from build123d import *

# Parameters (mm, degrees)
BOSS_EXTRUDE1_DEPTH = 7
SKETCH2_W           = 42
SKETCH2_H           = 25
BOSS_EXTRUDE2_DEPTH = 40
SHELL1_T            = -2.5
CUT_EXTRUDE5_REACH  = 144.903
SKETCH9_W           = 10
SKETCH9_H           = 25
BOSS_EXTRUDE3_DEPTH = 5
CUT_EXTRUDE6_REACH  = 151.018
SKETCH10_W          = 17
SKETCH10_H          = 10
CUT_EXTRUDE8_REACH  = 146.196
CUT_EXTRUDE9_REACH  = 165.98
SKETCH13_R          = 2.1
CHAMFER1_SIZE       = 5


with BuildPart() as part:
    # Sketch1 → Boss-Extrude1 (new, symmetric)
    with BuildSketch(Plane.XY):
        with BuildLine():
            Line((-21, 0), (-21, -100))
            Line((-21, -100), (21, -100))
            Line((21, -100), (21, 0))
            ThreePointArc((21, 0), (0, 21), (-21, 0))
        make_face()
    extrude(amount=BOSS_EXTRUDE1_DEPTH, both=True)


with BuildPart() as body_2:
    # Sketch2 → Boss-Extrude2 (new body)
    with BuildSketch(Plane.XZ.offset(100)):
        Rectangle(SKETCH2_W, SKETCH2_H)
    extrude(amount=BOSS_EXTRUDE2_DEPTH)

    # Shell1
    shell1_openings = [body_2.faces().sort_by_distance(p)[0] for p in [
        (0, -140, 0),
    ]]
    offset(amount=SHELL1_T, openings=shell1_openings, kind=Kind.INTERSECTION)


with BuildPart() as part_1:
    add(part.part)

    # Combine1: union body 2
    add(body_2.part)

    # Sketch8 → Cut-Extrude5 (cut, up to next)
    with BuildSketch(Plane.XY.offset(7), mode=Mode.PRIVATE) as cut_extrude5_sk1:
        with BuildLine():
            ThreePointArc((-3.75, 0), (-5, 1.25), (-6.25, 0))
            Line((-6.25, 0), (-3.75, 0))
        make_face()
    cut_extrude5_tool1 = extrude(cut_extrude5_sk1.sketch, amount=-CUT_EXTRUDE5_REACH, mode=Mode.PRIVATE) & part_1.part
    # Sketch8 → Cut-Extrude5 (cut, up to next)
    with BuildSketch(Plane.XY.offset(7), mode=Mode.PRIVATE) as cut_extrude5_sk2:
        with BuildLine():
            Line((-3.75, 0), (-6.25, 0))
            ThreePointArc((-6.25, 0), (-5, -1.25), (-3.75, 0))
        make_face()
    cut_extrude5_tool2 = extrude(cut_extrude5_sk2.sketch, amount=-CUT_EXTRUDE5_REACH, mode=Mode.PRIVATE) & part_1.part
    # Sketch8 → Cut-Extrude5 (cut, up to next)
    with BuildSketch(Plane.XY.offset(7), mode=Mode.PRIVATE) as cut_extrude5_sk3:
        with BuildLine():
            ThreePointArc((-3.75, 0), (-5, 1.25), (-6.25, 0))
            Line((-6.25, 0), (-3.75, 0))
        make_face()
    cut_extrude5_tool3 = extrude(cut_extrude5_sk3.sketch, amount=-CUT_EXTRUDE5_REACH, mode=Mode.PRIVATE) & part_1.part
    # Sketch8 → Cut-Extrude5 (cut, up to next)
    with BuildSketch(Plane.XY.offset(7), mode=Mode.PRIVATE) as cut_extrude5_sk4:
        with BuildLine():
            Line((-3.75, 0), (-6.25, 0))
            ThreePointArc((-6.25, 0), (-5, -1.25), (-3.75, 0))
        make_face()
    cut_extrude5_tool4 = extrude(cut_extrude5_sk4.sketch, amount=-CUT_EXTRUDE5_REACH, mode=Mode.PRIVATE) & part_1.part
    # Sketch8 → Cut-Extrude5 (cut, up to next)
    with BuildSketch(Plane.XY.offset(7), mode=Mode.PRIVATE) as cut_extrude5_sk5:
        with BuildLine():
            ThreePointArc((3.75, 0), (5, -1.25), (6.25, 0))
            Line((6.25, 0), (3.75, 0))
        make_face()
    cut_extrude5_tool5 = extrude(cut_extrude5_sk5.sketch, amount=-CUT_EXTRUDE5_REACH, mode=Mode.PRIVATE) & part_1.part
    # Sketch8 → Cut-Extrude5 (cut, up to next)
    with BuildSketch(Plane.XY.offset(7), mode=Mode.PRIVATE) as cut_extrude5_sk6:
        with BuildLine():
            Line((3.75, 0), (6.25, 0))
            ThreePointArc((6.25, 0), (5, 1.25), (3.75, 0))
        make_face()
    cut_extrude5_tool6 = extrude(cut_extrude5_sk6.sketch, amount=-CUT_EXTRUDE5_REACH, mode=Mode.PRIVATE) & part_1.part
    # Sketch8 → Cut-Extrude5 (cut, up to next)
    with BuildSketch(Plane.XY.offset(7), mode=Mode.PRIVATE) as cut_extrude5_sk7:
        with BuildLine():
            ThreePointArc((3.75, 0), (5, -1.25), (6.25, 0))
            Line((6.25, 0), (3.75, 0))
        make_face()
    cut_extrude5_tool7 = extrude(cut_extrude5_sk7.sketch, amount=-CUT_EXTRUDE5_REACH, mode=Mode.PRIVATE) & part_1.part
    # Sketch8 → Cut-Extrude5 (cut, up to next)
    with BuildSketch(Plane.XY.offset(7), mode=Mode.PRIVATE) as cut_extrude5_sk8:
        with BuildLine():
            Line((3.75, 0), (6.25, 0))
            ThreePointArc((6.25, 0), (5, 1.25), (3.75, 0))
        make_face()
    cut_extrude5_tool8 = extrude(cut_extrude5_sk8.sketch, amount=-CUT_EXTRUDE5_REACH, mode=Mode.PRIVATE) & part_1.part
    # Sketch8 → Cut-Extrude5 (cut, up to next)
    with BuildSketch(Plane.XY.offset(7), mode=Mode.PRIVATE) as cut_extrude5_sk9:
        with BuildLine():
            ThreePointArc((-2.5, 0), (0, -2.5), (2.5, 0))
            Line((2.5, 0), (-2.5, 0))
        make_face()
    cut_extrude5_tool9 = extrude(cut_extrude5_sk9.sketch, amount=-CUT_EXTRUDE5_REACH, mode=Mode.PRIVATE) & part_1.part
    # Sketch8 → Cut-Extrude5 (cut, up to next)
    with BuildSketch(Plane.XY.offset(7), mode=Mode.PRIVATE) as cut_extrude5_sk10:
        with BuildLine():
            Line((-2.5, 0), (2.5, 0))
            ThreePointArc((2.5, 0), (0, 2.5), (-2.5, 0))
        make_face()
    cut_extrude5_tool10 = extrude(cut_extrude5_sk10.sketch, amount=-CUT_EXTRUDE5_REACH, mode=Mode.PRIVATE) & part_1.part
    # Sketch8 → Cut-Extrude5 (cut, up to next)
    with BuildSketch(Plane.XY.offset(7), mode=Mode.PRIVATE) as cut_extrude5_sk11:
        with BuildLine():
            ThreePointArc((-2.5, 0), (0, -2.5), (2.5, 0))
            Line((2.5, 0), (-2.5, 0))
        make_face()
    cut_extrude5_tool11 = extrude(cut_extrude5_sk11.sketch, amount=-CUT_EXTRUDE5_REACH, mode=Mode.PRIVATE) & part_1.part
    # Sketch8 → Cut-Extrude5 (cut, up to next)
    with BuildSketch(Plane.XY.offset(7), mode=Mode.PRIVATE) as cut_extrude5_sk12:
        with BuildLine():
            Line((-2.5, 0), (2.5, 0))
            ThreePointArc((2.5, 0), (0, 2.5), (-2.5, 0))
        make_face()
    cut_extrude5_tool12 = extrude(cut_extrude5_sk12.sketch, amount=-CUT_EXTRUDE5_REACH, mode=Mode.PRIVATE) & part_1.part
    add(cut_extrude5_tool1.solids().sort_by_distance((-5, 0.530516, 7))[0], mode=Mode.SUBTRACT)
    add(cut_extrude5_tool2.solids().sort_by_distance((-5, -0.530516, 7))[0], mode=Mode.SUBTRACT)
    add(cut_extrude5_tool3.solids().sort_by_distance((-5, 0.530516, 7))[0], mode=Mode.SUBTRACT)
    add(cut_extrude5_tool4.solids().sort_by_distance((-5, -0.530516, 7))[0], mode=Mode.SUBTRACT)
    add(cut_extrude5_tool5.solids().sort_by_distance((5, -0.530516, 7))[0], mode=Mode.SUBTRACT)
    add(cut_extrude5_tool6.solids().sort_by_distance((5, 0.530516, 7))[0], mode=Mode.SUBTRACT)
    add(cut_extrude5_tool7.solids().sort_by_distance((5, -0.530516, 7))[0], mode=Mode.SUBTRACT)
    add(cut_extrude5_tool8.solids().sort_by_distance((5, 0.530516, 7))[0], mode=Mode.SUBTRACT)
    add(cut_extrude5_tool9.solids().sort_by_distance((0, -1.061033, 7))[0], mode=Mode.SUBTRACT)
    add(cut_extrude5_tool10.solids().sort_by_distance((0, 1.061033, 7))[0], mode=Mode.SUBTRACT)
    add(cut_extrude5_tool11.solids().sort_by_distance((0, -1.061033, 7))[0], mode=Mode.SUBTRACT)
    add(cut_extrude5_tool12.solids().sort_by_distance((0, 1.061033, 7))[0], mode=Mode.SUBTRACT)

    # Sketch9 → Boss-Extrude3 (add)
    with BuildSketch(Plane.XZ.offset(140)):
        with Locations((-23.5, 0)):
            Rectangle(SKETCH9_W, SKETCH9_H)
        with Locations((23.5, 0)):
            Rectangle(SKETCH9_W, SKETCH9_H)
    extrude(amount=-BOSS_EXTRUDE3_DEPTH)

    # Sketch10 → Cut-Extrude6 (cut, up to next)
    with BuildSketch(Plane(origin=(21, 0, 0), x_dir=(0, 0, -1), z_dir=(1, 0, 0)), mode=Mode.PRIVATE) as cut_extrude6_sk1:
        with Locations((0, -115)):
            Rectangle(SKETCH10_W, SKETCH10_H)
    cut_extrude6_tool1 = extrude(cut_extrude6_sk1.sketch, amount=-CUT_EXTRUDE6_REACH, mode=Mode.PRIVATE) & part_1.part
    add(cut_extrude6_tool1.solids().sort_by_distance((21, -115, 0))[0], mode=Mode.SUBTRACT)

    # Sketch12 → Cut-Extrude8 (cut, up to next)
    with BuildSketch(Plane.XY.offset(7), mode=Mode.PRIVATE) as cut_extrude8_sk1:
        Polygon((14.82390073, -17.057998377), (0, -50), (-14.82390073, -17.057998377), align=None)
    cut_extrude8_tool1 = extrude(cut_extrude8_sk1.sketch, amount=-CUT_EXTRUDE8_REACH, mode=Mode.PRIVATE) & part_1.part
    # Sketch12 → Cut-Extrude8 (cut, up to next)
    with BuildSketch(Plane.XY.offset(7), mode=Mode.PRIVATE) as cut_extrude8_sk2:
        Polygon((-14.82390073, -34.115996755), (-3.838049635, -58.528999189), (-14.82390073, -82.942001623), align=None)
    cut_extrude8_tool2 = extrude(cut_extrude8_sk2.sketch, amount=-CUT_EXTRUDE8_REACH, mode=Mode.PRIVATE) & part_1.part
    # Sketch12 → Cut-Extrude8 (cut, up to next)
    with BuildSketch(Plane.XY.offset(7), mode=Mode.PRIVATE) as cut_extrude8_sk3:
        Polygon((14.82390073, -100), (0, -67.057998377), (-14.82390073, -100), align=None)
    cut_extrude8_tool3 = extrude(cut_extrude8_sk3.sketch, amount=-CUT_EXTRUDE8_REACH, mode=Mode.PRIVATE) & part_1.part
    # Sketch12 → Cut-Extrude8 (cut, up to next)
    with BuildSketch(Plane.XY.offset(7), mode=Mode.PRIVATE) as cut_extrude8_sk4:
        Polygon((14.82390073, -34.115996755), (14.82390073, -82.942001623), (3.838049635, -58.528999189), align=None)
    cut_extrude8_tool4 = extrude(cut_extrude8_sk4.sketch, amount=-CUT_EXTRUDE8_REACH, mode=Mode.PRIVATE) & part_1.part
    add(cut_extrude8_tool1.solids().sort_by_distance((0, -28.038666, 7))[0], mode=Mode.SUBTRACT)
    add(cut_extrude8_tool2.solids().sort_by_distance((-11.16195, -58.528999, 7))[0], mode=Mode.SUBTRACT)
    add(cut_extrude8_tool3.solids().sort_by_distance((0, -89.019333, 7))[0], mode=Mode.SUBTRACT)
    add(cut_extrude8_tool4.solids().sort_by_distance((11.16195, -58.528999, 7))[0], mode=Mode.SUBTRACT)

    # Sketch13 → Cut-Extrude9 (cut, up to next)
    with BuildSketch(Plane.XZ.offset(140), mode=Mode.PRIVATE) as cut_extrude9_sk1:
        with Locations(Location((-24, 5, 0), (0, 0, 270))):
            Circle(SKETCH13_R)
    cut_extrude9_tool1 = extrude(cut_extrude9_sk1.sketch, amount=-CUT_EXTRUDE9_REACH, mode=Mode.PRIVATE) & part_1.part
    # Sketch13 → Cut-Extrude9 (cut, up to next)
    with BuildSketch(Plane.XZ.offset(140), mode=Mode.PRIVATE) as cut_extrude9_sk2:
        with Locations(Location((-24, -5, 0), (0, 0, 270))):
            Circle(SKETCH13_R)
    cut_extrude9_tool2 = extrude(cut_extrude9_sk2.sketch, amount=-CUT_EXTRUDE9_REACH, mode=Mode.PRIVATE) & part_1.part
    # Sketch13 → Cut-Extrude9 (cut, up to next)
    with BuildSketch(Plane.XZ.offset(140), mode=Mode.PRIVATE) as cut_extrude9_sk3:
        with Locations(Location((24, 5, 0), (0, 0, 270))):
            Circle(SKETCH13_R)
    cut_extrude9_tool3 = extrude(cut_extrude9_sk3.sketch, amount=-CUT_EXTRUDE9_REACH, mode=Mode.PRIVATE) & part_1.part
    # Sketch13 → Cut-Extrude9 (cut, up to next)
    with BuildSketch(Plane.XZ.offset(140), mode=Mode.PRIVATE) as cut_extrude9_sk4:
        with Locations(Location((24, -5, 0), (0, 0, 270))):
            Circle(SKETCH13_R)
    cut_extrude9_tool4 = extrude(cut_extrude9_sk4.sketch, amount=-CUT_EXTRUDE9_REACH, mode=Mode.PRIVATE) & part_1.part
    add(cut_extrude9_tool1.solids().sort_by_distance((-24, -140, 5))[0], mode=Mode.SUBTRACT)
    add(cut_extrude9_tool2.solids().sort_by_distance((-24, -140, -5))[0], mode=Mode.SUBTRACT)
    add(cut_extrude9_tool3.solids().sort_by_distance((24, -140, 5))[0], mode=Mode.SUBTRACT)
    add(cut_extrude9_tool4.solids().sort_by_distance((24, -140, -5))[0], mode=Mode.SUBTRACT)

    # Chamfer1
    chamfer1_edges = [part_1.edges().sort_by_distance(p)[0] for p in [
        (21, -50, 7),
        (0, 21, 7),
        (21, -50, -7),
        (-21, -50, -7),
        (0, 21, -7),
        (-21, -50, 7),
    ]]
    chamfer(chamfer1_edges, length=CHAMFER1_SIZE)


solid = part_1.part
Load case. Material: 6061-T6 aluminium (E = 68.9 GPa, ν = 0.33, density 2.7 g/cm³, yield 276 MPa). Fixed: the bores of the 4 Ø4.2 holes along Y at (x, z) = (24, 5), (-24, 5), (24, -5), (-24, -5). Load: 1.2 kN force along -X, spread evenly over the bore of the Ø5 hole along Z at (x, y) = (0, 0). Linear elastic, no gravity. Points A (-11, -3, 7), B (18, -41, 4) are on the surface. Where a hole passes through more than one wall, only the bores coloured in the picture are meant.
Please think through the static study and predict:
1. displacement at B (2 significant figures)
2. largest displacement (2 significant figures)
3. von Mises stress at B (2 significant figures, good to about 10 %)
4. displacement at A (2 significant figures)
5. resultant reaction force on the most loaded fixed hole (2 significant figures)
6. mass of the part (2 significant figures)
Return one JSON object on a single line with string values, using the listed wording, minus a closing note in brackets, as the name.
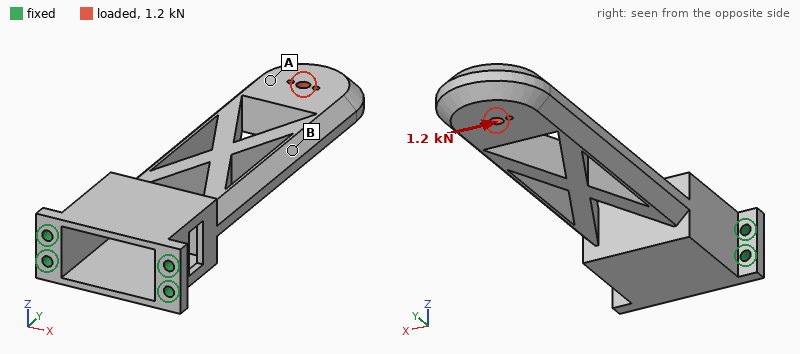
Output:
{"displacement at B": "0.31 mm", "largest displacement": "0.62 mm", "von Mises stress at B": "33 MPa", "displacement at A": "0.50 mm", "resultant reaction force on the most loaded fixed hole": "2.0 kN", "mass of the part": "150 g"}
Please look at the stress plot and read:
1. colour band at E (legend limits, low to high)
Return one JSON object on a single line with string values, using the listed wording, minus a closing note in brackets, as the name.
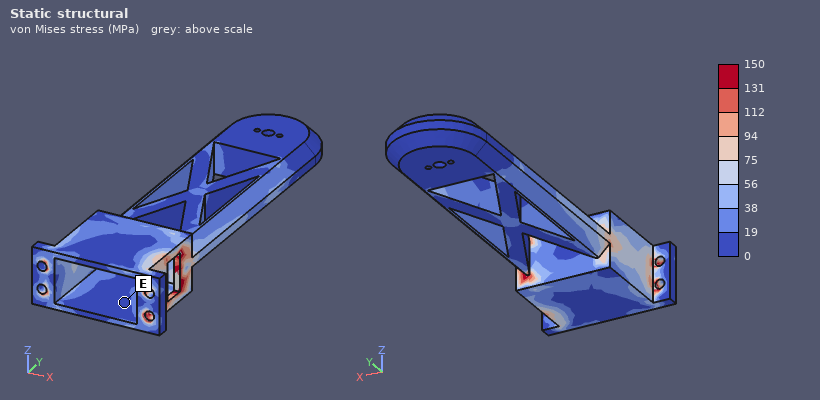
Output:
{"colour band at E": "0 to 19 MPa"}
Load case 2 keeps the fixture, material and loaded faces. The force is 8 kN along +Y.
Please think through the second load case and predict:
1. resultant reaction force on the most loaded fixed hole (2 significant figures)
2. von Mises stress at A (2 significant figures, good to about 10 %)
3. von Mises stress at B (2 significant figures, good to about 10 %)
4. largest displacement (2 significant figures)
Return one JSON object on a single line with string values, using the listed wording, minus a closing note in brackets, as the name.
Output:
{"resultant reaction force on the most loaded fixed hole": "2.1 kN", "von Mises stress at A": "21 MPa", "von Mises stress at B": "34 MPa", "largest displacement": "0.17 mm"}
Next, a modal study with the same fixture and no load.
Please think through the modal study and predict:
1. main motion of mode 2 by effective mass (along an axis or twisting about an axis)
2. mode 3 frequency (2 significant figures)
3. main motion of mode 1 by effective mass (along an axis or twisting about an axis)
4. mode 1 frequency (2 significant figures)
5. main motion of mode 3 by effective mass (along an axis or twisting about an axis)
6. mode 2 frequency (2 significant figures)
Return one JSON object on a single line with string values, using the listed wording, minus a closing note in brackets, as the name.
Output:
{"main motion of mode 2 by effective mass": "along X", "mode 3 frequency": "2100 Hz", "main motion of mode 1 by effective mass": "along Z", "mode 1 frequency": "360 Hz", "main motion of mode 3 by effective mass": "along Z", "mode 2 frequency": "990 Hz"}
